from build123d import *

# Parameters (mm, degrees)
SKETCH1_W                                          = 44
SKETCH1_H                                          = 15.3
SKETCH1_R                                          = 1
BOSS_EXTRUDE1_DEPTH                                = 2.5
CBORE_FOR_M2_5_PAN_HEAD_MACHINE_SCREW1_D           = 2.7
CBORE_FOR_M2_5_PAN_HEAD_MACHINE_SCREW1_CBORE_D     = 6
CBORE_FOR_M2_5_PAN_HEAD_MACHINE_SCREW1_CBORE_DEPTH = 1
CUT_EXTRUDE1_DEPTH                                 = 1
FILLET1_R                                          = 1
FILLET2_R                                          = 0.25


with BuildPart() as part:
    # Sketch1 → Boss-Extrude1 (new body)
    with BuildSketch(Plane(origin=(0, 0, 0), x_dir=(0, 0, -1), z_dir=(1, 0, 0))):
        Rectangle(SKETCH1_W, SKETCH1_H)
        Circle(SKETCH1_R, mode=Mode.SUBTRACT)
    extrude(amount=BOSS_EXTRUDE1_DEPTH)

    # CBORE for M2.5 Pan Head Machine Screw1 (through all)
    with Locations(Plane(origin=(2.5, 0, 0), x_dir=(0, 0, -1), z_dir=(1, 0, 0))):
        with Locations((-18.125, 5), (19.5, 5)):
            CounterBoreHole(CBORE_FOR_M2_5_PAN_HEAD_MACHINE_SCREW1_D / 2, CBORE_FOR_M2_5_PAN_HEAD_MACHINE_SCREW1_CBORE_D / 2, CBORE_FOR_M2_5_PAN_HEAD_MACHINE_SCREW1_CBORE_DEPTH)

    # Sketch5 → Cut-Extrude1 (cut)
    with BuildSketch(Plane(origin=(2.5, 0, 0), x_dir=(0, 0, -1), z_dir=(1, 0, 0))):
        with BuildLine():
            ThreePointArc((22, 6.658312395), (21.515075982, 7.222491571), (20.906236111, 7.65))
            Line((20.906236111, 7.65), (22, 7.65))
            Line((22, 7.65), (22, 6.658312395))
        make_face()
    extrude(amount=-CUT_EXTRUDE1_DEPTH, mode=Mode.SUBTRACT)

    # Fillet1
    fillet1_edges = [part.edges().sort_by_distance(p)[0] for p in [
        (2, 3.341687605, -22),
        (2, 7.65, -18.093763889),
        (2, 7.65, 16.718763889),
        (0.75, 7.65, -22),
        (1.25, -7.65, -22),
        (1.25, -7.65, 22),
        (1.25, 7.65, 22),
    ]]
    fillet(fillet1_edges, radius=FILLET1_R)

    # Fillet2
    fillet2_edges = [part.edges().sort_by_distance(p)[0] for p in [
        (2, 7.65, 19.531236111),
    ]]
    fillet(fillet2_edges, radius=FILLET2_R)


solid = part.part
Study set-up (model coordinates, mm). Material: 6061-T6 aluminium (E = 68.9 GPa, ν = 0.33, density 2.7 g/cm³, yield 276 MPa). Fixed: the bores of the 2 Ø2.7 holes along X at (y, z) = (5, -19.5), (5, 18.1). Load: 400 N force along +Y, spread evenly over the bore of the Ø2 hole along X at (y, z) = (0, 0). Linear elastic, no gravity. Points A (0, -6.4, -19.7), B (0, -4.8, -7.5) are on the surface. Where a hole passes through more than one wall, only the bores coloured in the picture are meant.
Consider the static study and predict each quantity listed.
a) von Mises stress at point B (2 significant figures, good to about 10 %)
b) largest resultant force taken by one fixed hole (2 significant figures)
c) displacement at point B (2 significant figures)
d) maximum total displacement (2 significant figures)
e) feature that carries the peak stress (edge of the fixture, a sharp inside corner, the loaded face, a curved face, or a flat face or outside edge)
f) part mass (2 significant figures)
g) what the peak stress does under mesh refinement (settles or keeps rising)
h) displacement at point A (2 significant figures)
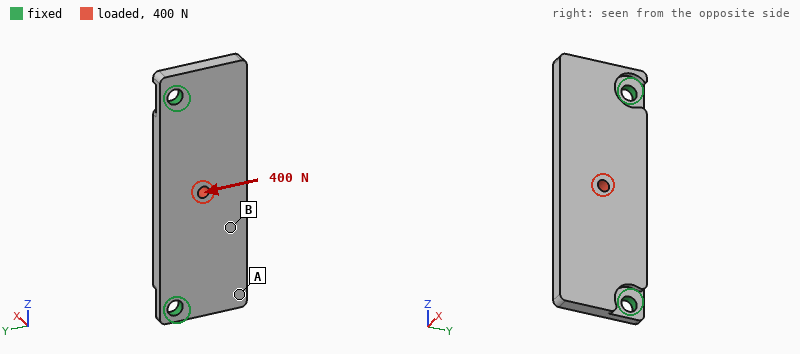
17 MPa
260 N
13 µm
17 µm
edge of the fixture
4.3 g
keeps rising
9.0 µm
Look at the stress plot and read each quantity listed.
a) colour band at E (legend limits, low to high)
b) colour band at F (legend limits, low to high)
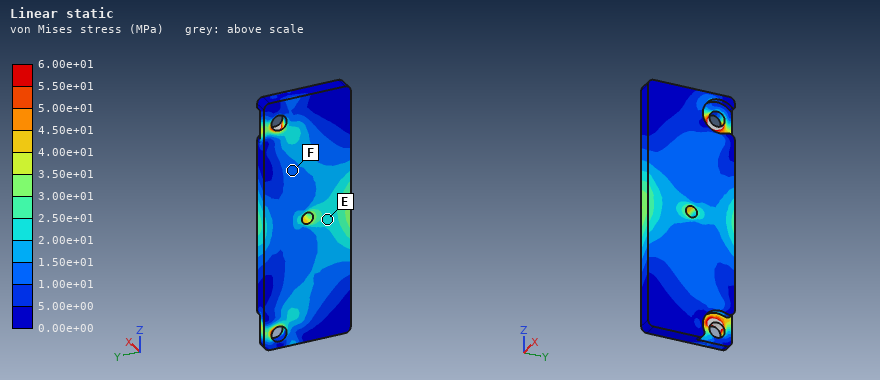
2.00e+01 to 2.50e+01 MPa
1.00e+01 to 1.50e+01 MPa
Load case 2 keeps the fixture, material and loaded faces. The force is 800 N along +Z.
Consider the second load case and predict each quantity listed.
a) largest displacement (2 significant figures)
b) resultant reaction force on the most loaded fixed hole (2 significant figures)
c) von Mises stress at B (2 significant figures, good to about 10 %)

7.8 µm
420 N
7.8 MPa
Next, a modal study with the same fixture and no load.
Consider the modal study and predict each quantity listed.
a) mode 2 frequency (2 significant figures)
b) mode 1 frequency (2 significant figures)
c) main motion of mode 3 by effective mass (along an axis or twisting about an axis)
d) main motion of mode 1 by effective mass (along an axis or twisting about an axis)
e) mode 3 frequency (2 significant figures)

9200 Hz
4700 Hz
twisting about Y
along X
11 kHz
